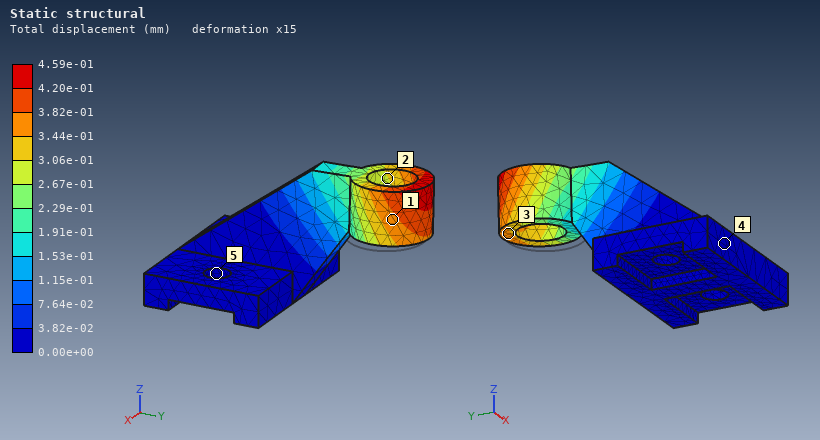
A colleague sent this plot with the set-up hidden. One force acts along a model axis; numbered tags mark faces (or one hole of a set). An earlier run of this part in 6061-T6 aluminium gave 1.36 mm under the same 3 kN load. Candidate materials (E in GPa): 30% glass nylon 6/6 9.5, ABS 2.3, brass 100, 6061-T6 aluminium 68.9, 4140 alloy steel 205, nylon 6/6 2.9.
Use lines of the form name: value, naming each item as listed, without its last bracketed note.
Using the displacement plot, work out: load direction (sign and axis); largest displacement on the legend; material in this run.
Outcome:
load direction: -X
largest displacement on the legend: 4.59e-01 mm
material in this run: 4140 alloy steel
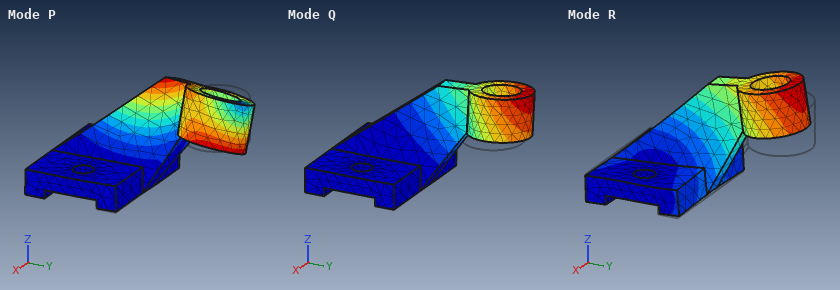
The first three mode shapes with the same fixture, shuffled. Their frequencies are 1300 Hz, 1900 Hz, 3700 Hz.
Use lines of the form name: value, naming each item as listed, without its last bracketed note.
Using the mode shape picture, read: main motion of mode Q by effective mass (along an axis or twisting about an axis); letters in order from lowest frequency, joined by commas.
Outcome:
main motion of mode Q by effective mass: along X
letters in order from lowest frequency, joined by commas: Q, R, P
